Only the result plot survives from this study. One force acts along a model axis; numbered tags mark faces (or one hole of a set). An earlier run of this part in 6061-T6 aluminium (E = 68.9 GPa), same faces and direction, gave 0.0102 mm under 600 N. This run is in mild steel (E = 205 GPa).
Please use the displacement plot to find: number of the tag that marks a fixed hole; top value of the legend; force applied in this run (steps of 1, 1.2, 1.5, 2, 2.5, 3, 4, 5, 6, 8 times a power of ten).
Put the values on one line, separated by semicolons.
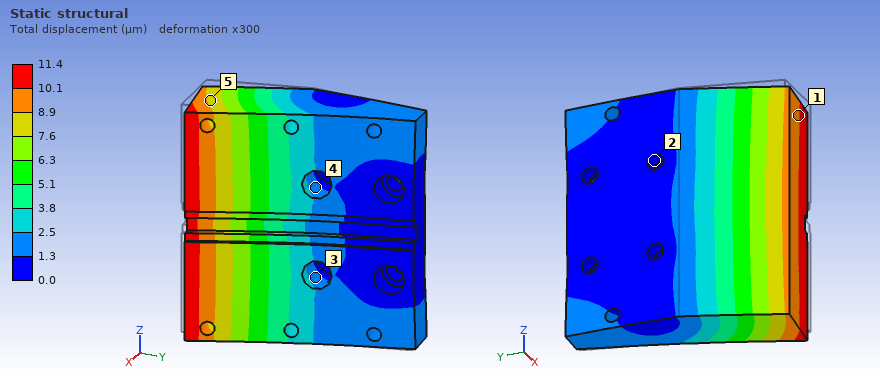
2; 11.4 µm; 2 kN
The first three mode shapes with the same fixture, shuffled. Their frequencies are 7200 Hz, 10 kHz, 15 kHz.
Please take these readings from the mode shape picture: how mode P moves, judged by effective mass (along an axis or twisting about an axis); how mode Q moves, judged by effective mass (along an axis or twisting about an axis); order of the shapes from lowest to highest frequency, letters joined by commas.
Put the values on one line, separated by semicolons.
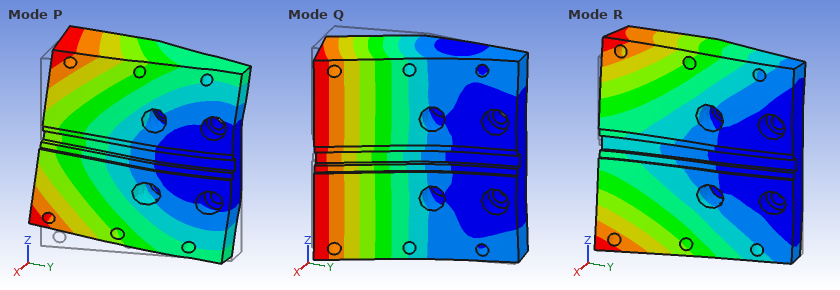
along Z; along X; Q, R, P
